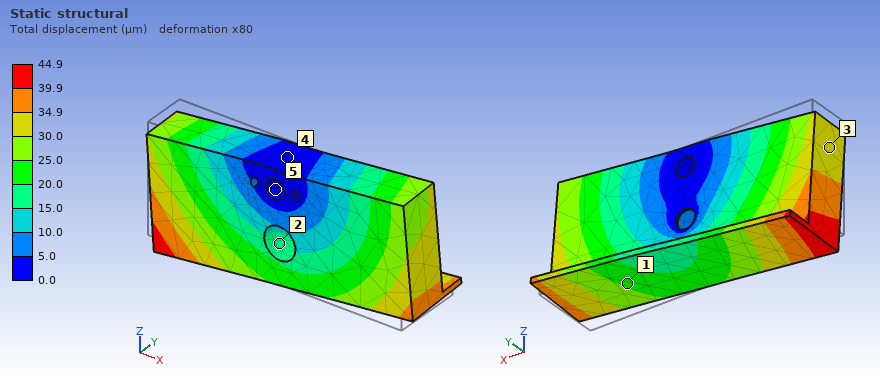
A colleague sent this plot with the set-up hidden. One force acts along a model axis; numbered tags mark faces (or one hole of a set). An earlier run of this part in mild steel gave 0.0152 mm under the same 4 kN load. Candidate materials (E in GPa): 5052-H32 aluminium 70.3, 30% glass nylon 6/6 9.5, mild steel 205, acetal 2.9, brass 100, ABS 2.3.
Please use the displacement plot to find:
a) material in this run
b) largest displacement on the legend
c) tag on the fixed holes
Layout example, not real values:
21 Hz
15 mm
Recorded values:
5052-H32 aluminium
44.9 µm
5
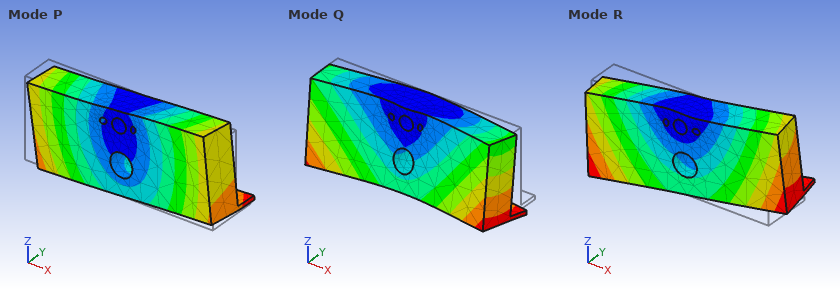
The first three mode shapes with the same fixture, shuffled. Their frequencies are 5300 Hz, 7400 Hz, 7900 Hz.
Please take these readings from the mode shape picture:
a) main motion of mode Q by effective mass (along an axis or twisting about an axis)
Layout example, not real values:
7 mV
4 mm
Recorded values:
along Y
